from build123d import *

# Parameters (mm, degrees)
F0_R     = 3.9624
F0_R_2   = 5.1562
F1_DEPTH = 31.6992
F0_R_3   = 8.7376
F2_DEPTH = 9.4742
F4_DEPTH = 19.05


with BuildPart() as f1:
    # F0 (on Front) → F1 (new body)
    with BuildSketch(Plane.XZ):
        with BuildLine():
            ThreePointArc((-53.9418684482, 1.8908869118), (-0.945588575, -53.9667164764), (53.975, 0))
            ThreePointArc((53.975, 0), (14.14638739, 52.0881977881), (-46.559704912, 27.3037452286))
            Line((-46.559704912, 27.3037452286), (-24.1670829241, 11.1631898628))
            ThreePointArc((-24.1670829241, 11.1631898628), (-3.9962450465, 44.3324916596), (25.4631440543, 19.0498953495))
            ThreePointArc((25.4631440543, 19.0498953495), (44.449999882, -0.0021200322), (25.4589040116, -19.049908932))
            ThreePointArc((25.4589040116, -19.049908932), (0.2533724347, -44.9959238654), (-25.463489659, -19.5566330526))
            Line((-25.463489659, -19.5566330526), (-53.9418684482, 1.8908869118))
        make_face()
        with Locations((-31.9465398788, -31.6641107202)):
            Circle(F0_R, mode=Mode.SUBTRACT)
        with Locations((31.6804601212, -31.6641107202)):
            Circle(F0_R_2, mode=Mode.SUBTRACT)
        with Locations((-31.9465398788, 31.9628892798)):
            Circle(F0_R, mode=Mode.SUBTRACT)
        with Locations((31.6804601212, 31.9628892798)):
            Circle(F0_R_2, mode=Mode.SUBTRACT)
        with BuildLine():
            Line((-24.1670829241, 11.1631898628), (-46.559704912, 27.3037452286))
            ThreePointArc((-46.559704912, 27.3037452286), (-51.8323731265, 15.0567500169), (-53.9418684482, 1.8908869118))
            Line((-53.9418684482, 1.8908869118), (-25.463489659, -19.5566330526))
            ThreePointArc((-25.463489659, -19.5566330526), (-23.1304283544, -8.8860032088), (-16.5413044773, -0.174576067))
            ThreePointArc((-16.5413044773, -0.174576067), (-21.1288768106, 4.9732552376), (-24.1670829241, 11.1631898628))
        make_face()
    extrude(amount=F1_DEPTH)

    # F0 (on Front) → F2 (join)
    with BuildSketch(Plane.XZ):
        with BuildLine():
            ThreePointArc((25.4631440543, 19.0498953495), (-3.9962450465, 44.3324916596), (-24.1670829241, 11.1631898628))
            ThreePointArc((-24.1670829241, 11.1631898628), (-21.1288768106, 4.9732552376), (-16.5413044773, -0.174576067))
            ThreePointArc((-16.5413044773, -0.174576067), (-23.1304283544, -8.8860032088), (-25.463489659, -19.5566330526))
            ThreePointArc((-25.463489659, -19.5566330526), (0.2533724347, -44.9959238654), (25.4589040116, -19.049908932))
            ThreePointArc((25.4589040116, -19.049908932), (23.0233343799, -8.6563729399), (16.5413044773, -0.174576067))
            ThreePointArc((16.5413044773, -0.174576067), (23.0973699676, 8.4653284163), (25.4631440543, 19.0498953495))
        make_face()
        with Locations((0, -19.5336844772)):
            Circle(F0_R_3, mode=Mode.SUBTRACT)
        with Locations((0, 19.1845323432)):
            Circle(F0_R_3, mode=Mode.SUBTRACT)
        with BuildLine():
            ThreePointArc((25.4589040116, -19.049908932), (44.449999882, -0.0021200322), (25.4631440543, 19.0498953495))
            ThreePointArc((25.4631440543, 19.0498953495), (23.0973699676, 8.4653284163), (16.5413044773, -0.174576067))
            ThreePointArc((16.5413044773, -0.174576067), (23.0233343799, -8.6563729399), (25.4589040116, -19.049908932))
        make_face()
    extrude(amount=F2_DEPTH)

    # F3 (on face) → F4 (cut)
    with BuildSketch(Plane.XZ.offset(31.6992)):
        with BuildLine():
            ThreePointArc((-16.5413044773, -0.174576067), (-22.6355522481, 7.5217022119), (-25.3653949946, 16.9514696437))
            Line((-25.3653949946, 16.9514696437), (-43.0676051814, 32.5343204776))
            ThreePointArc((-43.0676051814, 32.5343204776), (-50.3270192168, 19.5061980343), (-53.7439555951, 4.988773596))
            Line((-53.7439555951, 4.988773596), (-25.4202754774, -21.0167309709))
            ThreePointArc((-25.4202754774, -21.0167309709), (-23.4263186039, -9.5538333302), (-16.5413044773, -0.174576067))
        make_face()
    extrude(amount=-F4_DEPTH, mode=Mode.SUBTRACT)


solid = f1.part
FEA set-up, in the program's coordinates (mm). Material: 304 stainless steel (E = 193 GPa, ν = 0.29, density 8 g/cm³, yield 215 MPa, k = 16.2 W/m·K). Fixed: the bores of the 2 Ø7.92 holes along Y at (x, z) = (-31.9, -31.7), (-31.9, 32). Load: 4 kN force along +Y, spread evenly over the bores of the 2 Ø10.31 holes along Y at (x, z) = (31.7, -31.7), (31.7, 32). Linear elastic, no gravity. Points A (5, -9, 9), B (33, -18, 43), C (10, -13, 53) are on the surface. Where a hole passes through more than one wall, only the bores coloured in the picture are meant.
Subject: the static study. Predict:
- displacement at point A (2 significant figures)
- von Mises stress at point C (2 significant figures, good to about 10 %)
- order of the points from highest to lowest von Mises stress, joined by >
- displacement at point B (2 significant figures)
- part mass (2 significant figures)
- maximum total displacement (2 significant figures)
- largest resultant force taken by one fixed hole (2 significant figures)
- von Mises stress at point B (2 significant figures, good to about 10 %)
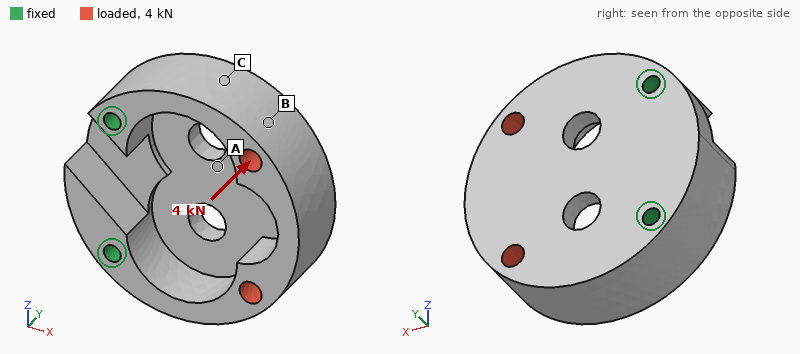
20 µm
17 MPa
B > C > A
39 µm
1.3 kg
68 µm
2.1 kN
24 MPa
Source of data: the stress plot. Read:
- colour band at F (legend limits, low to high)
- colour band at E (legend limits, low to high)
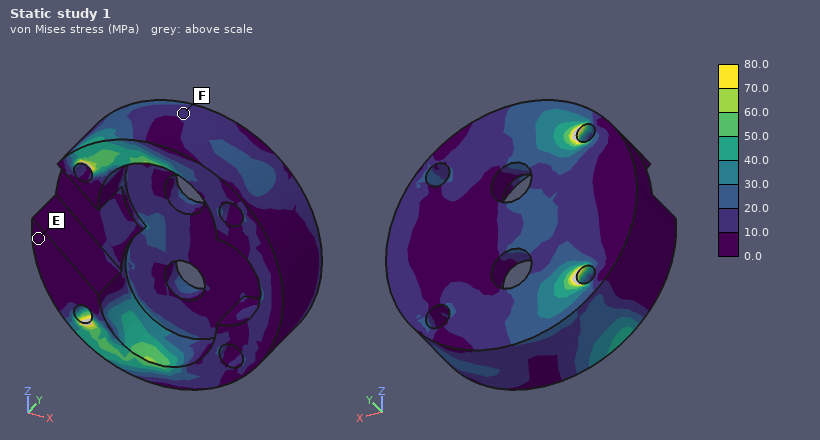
10.0 to 20.0 MPa
0.0 to 10.0 MPa
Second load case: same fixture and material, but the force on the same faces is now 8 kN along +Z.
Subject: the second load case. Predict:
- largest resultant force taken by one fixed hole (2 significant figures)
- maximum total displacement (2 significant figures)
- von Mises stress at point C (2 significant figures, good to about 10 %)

7.9 kN
33 µm
17 MPa
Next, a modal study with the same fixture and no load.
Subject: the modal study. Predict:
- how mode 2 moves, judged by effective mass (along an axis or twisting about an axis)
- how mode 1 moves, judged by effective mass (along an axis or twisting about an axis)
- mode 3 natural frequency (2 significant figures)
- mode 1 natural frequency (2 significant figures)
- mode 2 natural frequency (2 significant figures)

along Z
along Y
5600 Hz
1900 Hz
3800 Hz
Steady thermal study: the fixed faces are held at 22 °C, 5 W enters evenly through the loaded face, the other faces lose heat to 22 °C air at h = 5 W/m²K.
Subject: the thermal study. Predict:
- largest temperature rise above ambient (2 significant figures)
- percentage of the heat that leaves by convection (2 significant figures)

14 K
23 %
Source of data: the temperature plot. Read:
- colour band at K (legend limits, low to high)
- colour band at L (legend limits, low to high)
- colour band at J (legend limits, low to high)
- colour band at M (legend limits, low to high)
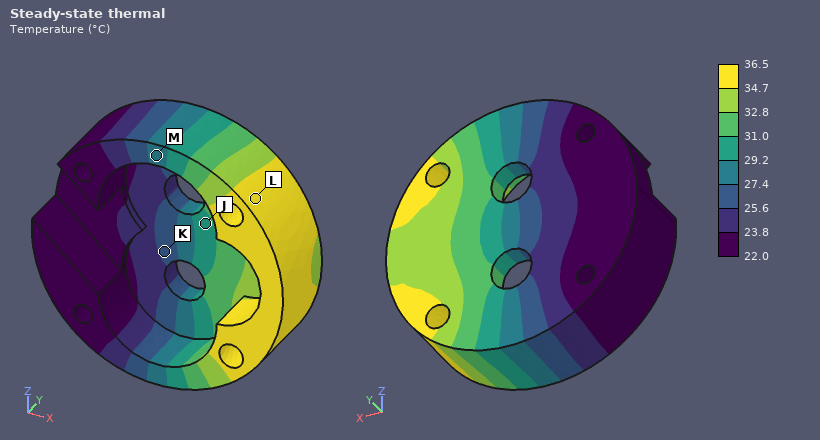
25.6 to 27.4 °C
34.7 to 36.5 °C
29.2 to 31.0 °C
27.4 to 29.2 °C
